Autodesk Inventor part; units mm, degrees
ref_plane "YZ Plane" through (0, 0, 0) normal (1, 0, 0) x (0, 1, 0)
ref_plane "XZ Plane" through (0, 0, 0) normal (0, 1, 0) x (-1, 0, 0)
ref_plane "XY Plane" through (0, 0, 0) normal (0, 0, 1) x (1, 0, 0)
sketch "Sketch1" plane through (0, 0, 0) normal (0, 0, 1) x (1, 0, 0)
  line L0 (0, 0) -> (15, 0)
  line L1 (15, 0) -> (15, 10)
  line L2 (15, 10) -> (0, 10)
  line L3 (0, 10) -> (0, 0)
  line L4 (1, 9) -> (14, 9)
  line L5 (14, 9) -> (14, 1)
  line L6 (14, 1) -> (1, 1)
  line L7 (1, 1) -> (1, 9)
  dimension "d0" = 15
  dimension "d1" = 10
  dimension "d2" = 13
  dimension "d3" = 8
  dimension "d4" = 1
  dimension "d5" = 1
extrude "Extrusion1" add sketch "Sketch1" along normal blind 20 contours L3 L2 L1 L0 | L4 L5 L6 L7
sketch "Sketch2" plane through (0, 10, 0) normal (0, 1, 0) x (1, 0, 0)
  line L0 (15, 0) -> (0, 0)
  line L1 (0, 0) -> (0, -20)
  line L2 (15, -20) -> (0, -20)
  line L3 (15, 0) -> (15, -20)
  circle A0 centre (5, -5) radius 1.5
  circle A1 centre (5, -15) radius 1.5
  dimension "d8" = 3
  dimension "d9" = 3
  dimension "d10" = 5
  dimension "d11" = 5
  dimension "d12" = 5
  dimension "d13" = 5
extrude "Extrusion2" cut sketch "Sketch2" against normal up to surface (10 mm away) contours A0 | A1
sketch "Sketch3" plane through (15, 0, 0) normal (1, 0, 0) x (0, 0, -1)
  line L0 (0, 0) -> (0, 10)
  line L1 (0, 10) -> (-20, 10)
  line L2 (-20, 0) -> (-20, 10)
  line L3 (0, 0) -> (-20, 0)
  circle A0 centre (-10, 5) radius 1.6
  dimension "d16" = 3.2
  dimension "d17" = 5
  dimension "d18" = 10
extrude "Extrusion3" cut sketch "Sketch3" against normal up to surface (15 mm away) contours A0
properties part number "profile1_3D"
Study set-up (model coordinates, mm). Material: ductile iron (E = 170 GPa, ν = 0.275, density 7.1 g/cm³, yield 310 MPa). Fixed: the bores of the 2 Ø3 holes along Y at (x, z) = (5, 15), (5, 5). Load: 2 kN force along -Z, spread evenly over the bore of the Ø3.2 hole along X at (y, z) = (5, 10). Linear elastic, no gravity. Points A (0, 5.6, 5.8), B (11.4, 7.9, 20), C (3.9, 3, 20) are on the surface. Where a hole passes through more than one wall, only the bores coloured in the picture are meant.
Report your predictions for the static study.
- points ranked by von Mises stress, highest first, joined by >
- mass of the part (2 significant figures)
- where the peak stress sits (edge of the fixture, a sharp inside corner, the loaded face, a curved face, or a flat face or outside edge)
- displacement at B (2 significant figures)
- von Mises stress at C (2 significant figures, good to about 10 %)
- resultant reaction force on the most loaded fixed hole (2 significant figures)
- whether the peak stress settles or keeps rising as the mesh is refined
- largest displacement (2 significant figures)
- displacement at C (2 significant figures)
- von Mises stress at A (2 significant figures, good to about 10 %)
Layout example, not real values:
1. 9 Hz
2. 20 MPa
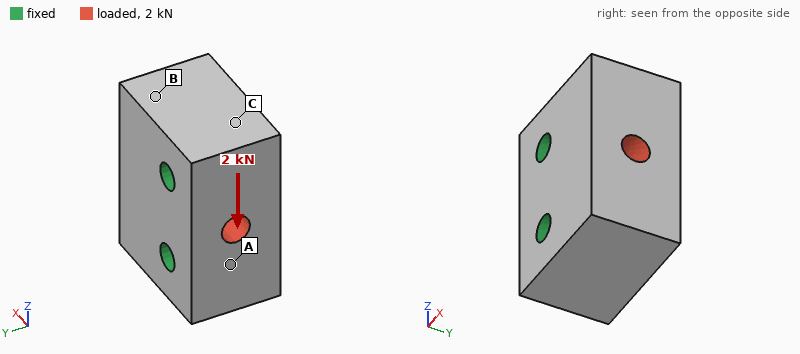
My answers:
1. A > C > B
2. 19 g
3. edge of the fixture
4. 0.69 µm
5. 5.9 MPa
6. 1.1 kN
7. keeps rising
8. 1.0 µm
9. 0.18 µm
10. 9.2 MPa
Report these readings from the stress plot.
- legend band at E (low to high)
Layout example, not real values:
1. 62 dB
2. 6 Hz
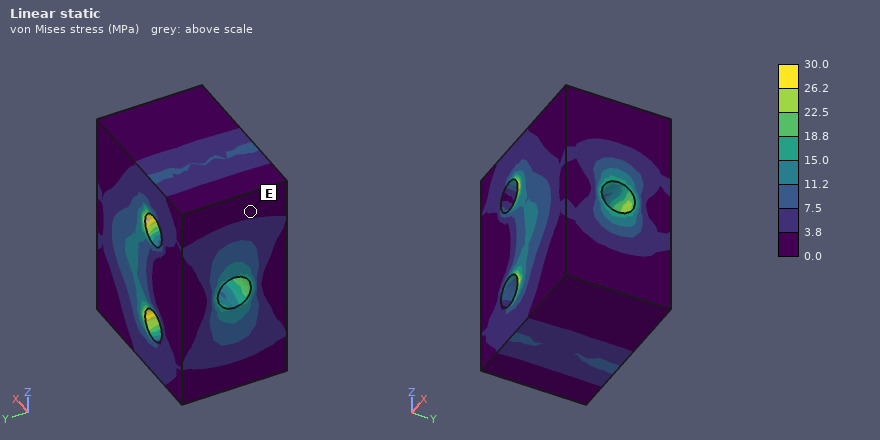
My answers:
1. 0.0 to 3.8 MPa
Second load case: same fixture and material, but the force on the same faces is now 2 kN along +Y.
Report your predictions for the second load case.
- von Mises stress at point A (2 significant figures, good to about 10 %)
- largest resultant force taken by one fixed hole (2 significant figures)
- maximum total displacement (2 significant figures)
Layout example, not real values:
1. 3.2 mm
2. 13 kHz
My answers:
1. 6.2 MPa
2. 1.0 kN
3. 1.8 µm
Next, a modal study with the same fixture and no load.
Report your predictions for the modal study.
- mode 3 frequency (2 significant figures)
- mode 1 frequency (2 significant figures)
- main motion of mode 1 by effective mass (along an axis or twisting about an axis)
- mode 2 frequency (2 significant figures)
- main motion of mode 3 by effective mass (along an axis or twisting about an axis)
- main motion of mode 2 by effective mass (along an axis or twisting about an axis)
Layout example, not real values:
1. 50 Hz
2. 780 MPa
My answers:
1. 64 kHz
2. 51 kHz
3. along Y
4. 56 kHz
5. twisting about X
6. along Z
